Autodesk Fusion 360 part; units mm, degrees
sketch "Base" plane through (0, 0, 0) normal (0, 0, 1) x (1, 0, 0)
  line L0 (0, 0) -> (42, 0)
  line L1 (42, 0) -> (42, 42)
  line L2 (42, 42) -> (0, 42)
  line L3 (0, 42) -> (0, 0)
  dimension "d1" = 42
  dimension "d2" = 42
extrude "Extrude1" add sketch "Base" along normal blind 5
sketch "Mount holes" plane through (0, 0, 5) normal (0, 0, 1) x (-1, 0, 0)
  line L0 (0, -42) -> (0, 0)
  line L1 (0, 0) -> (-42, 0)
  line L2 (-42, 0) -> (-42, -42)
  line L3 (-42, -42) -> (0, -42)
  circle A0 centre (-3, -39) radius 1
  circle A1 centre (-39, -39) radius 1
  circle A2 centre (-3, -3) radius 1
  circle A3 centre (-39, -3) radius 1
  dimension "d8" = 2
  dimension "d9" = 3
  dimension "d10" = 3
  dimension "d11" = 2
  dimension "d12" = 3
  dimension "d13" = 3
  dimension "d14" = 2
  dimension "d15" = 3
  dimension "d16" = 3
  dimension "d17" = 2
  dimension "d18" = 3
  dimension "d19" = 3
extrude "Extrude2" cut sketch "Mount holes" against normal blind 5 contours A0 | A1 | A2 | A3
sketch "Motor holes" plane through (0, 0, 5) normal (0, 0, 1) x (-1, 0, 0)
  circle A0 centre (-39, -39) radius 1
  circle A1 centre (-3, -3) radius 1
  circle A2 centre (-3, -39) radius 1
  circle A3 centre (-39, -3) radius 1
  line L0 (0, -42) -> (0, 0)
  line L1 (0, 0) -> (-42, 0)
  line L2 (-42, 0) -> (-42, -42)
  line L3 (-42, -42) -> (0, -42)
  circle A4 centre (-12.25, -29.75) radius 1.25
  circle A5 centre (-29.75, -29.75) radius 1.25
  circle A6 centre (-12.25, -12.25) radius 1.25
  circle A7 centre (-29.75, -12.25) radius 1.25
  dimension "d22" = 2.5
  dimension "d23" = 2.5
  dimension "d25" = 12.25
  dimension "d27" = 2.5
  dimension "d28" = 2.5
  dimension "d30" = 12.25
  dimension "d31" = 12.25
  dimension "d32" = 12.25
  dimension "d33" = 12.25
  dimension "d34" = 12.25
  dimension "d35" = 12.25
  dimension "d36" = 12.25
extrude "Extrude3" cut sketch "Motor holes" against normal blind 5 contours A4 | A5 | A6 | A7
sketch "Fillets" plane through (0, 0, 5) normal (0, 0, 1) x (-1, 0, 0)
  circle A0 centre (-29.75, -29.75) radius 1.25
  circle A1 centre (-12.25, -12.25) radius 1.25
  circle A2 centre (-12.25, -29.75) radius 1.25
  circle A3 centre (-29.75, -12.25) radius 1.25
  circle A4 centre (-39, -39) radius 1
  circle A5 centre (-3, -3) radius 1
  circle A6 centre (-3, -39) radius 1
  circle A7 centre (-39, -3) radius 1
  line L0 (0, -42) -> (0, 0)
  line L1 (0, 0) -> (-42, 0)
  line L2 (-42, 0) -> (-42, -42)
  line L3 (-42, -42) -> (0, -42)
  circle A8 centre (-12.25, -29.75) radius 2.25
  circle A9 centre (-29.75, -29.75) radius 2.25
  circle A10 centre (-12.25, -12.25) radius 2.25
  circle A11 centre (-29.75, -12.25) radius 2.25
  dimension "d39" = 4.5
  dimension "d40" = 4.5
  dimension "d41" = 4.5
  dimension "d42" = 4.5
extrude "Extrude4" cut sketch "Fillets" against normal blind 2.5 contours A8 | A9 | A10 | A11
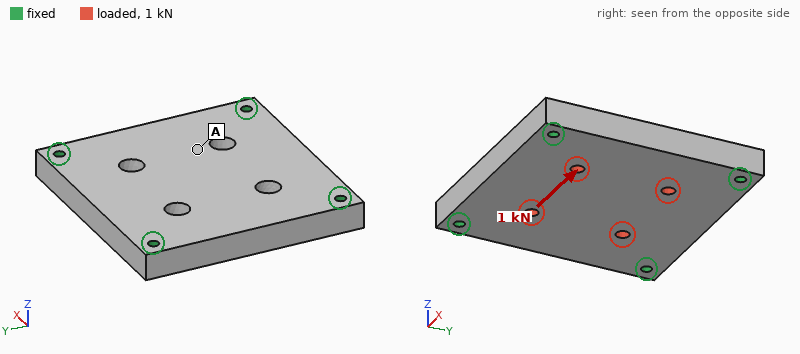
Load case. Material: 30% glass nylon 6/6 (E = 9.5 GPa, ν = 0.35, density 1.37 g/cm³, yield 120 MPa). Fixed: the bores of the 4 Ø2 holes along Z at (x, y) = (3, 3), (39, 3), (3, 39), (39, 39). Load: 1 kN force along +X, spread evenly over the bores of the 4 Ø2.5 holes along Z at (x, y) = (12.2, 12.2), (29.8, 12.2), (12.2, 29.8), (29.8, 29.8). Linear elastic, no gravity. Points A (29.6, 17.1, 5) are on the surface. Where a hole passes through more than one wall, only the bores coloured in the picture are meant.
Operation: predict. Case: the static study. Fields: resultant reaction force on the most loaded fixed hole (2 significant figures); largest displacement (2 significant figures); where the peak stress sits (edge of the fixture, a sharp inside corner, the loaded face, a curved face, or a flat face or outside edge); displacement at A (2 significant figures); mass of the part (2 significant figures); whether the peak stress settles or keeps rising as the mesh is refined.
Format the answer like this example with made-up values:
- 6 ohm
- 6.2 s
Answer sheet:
- 270 N
- 16 µm
- edge of the fixture
- 11 µm
- 12 g
- keeps rising
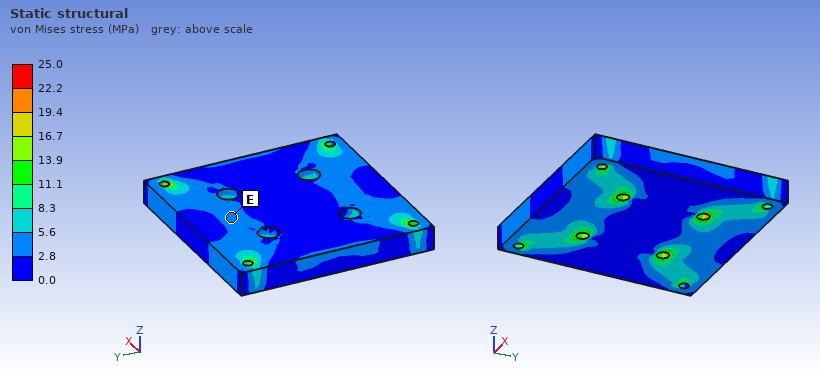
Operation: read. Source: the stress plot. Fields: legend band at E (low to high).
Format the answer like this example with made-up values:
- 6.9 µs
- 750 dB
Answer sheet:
- 2.8 to 5.6 MPa
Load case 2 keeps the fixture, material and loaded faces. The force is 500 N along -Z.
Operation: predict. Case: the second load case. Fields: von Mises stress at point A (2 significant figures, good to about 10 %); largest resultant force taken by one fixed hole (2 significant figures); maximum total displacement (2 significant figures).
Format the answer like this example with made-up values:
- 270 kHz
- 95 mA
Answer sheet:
- 8.4 MPa
- 130 N
- 65 µm
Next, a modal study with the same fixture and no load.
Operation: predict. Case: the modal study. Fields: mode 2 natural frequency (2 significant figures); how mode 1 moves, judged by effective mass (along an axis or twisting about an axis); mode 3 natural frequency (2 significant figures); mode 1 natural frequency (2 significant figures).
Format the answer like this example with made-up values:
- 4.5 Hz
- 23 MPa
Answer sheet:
- 9600 Hz
- along Z
- 9600 Hz
- 5800 Hz
